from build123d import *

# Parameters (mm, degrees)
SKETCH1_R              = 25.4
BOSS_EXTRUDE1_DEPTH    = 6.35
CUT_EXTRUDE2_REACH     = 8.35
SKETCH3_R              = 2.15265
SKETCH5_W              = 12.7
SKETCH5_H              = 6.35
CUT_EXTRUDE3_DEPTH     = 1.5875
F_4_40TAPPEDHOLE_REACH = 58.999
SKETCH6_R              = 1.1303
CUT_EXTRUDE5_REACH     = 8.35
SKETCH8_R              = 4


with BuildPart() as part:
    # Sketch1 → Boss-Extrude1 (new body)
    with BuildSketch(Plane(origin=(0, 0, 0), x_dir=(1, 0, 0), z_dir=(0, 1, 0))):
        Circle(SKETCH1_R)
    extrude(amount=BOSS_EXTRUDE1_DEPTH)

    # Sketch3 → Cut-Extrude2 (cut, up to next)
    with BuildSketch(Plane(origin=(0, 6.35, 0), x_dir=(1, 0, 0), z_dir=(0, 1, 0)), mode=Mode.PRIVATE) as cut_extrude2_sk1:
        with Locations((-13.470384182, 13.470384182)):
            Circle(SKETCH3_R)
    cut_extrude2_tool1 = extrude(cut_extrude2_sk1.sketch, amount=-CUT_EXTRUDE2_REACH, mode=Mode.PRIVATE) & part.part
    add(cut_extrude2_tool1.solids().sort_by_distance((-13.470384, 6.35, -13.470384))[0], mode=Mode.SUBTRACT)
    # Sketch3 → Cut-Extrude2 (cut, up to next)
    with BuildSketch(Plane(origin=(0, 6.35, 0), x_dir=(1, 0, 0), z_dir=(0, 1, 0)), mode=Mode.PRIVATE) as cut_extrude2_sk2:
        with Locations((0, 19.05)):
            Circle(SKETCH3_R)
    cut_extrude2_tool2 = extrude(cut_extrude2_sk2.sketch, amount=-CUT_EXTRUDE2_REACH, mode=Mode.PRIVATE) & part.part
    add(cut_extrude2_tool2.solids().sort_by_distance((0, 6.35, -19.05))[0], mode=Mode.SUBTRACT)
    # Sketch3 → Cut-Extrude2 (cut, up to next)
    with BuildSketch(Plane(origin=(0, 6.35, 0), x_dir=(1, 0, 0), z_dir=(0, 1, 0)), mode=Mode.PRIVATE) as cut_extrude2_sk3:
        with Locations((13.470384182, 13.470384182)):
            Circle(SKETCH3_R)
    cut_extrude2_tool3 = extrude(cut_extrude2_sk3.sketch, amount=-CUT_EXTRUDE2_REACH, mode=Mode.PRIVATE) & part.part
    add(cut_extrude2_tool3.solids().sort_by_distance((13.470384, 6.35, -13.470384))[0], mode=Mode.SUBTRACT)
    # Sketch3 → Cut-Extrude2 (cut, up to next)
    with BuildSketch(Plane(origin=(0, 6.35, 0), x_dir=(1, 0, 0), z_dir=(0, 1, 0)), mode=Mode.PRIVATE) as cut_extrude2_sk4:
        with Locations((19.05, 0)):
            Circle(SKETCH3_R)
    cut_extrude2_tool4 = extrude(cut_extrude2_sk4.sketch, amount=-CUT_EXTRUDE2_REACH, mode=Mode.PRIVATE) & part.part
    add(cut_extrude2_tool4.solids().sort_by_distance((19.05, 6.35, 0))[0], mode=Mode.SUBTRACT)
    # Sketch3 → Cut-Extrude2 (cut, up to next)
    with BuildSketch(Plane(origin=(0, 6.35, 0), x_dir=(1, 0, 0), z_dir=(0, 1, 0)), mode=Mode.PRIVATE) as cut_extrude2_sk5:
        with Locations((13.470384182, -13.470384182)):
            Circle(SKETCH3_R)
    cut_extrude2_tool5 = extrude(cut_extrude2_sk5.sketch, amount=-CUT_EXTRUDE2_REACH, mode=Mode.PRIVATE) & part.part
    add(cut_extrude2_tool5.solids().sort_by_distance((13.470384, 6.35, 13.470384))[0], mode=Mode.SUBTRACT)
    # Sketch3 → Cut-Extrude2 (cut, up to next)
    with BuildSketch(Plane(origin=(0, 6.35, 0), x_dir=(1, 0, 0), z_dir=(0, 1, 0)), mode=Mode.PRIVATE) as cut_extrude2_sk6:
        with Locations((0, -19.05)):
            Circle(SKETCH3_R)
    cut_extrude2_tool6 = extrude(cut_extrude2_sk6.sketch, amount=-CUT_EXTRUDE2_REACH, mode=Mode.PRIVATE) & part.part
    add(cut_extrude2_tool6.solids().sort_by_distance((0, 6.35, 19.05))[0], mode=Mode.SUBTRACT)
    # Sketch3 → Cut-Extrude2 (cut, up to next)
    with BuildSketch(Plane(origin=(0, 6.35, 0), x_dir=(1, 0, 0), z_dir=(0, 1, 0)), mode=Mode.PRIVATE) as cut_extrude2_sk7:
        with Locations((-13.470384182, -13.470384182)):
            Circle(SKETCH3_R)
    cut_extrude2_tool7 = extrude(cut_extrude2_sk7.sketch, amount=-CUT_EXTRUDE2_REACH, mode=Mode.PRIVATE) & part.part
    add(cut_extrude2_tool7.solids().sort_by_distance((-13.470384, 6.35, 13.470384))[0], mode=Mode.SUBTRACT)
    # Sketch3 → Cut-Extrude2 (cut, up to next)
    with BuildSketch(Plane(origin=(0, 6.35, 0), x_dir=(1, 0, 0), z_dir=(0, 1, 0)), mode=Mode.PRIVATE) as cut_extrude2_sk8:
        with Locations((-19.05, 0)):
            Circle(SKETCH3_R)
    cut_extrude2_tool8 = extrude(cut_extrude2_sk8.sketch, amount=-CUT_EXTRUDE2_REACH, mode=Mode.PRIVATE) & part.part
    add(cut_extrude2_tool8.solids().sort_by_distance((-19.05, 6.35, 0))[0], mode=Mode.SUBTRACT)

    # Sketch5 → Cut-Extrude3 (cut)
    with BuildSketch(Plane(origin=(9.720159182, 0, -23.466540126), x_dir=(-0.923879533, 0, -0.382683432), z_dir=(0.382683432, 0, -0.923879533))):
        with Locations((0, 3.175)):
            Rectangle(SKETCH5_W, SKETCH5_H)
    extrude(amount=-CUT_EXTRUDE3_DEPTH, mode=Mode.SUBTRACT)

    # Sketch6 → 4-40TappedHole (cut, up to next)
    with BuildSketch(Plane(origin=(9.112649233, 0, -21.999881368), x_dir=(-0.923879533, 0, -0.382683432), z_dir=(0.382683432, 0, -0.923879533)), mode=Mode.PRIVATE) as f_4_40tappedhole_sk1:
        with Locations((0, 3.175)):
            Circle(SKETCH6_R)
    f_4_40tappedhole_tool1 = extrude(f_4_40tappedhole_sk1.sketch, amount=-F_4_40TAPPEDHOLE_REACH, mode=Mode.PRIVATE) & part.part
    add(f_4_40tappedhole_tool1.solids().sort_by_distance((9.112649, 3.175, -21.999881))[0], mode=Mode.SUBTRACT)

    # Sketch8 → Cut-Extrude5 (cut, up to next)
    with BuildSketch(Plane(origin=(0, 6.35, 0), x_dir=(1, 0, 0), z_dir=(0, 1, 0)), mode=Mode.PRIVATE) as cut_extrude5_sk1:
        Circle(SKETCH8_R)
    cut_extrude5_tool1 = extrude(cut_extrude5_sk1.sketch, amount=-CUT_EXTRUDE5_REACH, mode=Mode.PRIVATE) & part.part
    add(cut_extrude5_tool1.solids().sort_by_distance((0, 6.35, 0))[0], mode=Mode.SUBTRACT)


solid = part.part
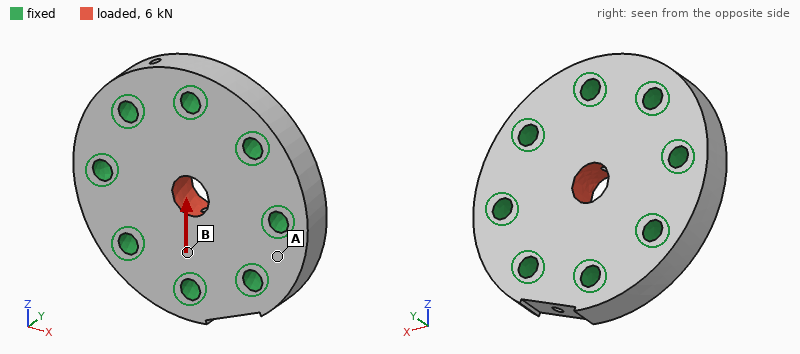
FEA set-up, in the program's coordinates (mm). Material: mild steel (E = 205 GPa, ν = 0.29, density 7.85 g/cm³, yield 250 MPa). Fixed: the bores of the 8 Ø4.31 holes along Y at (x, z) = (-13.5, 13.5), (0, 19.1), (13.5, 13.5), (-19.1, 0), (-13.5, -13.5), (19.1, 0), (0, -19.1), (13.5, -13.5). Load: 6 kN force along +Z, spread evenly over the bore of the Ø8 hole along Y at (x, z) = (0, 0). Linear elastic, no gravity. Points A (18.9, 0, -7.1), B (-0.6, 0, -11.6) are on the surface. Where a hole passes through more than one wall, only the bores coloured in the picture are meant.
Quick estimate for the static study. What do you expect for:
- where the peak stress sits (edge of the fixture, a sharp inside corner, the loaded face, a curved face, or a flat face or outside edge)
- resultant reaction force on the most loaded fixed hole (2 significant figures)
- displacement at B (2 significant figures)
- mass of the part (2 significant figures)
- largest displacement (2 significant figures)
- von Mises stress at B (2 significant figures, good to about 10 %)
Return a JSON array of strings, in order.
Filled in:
["the loaded face", "1.3 kN", "0.68 µm", "91 g", "2.0 µm", "25 MPa"]
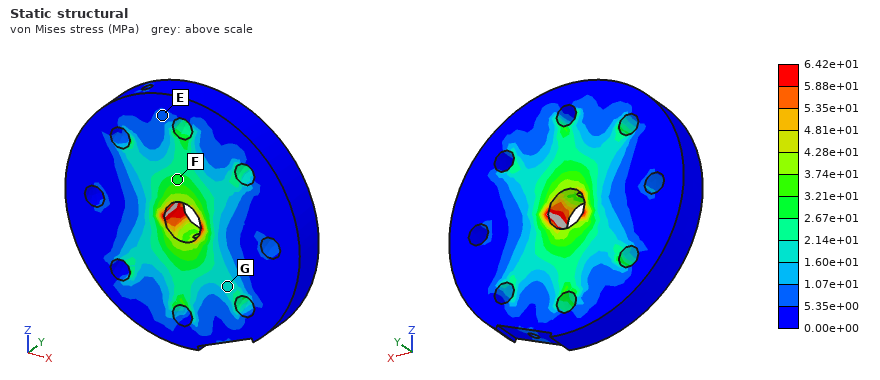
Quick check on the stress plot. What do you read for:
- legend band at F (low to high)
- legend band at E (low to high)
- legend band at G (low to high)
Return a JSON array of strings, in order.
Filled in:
["2.67e+01 to 3.21e+01 MPa", "5.35e+00 to 1.07e+01 MPa", "1.60e+01 to 2.14e+01 MPa"]
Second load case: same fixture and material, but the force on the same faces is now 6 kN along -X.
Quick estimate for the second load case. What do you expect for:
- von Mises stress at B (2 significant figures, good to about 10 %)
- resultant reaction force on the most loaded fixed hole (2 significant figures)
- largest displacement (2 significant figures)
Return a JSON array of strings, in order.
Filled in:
["5.9 MPa", "1.3 kN", "2.0 µm"]
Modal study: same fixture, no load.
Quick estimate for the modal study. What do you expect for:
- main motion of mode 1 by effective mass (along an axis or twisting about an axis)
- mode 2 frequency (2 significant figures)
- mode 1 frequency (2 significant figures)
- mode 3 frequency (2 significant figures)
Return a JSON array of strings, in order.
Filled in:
["along Y", "58 kHz", "37 kHz", "61 kHz"]
